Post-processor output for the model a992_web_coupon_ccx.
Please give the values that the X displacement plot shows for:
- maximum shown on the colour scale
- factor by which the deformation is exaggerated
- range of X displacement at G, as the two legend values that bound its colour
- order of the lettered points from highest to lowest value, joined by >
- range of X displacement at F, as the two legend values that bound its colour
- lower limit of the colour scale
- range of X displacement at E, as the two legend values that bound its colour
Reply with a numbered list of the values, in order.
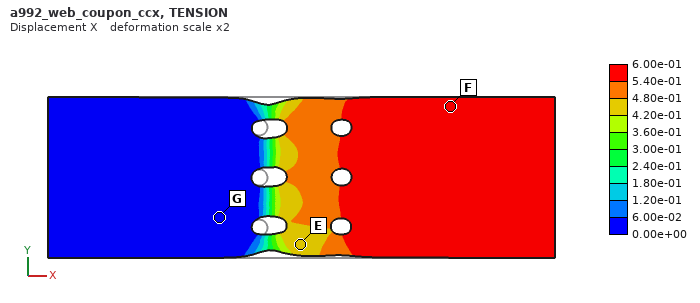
1. 6.00e-01
2. 2
3. 0.00e+00 to 6.00e-02
4. F > E > G
5. 5.40e-01 to 6.00e-01
6. 0.00e+00
7. 4.20e-01 to 4.80e-01
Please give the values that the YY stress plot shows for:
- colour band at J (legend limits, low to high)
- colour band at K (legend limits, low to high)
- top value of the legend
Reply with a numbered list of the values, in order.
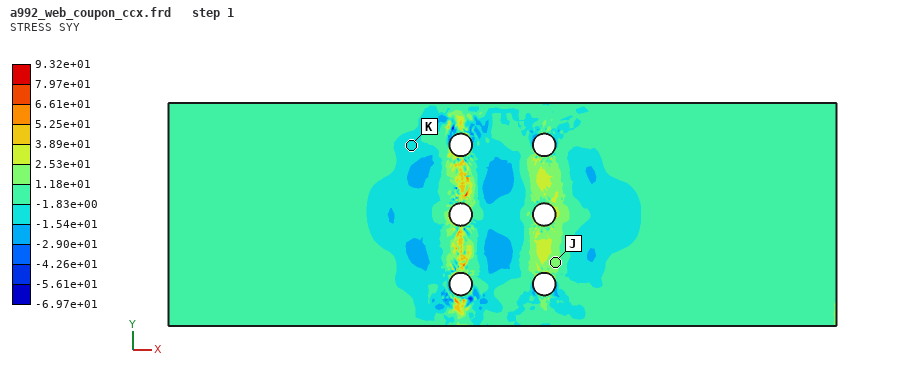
1. 1.18e+01 to 2.53e+01
2. -1.54e+01 to -1.83e+00
3. 9.32e+01
